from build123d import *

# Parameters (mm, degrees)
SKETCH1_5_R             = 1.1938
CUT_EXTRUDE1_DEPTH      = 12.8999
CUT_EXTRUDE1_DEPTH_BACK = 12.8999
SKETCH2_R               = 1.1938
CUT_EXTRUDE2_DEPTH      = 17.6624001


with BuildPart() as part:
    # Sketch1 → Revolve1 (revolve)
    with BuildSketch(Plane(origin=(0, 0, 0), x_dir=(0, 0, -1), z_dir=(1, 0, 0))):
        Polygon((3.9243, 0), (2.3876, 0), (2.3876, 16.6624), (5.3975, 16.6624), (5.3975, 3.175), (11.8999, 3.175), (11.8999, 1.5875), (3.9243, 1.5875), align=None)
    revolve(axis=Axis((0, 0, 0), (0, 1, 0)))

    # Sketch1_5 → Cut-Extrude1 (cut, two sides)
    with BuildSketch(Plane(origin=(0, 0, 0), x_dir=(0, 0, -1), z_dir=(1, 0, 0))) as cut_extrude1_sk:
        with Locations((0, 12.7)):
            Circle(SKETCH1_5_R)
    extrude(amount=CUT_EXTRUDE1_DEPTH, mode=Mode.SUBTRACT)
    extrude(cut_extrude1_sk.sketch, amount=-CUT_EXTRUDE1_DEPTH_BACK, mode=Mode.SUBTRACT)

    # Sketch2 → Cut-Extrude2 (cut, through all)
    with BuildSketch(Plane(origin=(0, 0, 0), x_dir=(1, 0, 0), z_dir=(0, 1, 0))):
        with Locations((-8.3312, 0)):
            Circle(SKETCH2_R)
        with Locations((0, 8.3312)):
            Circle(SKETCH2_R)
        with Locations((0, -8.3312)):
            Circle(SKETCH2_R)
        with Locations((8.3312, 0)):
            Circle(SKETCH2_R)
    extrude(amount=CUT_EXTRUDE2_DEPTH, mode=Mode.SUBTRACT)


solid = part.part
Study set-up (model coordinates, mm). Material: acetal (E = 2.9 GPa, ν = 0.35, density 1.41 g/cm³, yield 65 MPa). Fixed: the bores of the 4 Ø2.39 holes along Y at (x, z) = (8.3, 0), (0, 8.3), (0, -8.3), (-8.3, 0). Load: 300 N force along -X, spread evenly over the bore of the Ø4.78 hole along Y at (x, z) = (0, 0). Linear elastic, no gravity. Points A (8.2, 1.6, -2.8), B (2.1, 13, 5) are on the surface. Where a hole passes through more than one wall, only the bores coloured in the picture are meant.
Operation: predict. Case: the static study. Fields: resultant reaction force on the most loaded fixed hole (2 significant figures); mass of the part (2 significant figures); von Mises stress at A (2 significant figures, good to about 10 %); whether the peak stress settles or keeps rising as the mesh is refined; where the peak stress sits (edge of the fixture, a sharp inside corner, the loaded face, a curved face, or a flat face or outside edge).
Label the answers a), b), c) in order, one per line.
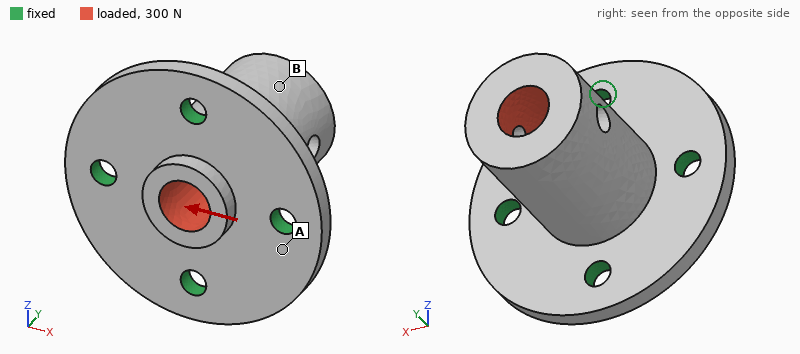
a) 160 N
b) 2.3 g
c) 11 MPa
d) keeps rising
e) edge of the fixture
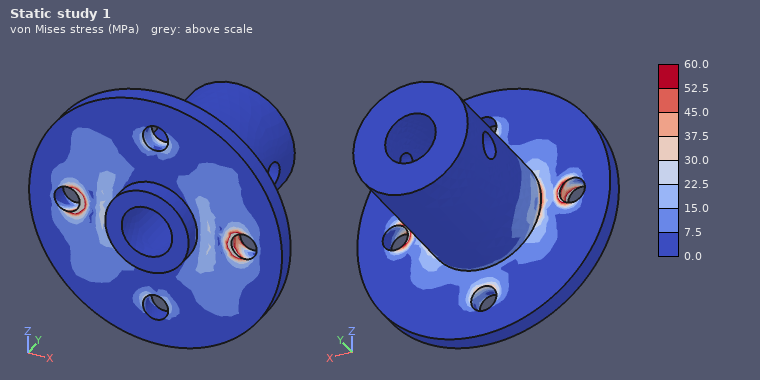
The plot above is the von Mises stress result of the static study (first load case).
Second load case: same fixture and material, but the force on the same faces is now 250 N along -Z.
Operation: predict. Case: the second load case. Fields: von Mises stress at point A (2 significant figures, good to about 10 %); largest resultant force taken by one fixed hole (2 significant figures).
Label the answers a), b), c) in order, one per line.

a) 5.1 MPa
b) 130 N
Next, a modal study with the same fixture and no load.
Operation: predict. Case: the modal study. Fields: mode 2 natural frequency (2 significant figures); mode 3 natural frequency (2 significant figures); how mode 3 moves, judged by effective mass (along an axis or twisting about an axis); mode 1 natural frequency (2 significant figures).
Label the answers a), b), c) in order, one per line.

a) 4800 Hz
b) 8900 Hz
c) along Y
d) 4700 Hz
